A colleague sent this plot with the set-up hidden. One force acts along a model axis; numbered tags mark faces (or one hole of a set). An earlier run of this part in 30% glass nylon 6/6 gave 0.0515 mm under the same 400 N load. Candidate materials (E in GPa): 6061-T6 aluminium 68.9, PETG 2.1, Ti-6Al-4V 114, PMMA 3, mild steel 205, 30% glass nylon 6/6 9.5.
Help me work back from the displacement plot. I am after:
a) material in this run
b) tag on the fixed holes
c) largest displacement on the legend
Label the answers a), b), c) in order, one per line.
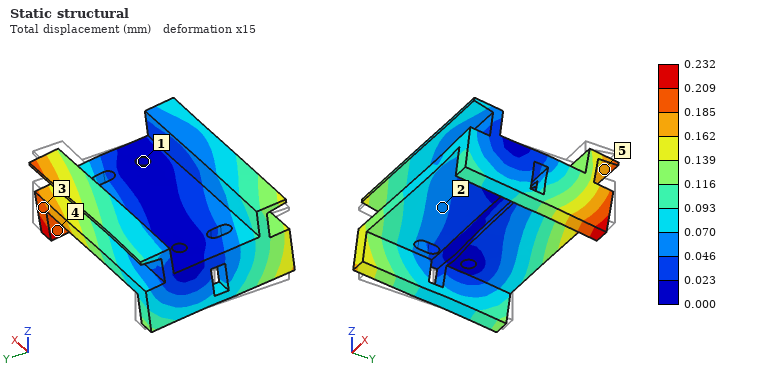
a) PETG
b) 1
c) 0.232 mm
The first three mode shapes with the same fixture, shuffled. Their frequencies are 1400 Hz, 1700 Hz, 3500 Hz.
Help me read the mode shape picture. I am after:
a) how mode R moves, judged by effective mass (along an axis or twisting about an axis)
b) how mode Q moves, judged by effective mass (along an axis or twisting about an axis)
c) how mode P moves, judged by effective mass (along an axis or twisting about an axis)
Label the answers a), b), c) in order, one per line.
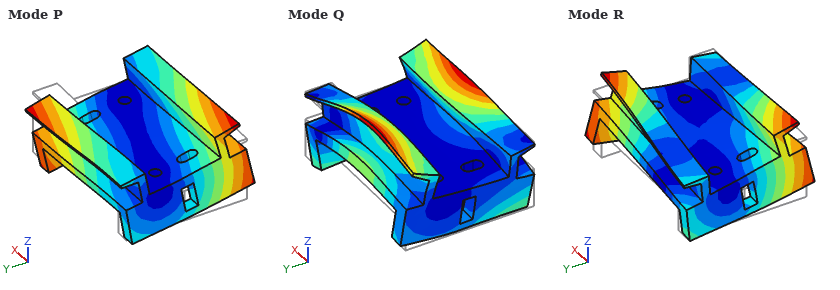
a) along Z
b) along Z
c) twisting about X
